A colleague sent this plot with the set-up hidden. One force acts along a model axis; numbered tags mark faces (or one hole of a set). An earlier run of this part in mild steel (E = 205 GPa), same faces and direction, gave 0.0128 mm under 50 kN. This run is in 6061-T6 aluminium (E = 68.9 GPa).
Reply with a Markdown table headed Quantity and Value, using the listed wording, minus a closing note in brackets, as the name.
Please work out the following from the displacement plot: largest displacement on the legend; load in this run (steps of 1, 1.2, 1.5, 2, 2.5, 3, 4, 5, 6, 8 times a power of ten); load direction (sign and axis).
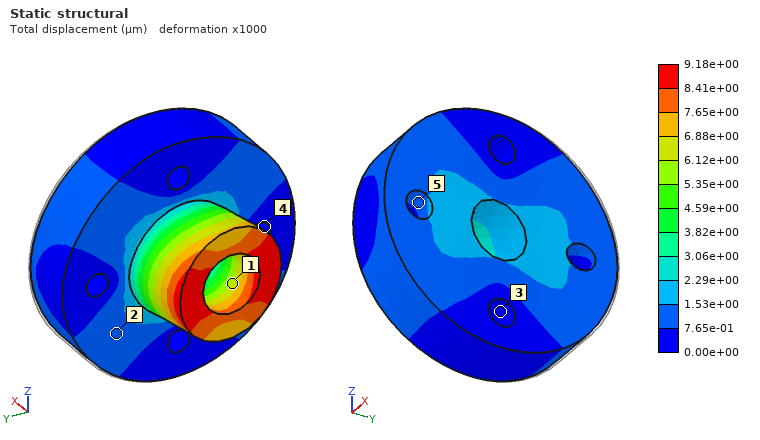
| Quantity | Value |
|---|---|
| largest displacement on the legend | 9.18e+00 µm |
| load in this run | 12 kN |
| load direction | -Y |
